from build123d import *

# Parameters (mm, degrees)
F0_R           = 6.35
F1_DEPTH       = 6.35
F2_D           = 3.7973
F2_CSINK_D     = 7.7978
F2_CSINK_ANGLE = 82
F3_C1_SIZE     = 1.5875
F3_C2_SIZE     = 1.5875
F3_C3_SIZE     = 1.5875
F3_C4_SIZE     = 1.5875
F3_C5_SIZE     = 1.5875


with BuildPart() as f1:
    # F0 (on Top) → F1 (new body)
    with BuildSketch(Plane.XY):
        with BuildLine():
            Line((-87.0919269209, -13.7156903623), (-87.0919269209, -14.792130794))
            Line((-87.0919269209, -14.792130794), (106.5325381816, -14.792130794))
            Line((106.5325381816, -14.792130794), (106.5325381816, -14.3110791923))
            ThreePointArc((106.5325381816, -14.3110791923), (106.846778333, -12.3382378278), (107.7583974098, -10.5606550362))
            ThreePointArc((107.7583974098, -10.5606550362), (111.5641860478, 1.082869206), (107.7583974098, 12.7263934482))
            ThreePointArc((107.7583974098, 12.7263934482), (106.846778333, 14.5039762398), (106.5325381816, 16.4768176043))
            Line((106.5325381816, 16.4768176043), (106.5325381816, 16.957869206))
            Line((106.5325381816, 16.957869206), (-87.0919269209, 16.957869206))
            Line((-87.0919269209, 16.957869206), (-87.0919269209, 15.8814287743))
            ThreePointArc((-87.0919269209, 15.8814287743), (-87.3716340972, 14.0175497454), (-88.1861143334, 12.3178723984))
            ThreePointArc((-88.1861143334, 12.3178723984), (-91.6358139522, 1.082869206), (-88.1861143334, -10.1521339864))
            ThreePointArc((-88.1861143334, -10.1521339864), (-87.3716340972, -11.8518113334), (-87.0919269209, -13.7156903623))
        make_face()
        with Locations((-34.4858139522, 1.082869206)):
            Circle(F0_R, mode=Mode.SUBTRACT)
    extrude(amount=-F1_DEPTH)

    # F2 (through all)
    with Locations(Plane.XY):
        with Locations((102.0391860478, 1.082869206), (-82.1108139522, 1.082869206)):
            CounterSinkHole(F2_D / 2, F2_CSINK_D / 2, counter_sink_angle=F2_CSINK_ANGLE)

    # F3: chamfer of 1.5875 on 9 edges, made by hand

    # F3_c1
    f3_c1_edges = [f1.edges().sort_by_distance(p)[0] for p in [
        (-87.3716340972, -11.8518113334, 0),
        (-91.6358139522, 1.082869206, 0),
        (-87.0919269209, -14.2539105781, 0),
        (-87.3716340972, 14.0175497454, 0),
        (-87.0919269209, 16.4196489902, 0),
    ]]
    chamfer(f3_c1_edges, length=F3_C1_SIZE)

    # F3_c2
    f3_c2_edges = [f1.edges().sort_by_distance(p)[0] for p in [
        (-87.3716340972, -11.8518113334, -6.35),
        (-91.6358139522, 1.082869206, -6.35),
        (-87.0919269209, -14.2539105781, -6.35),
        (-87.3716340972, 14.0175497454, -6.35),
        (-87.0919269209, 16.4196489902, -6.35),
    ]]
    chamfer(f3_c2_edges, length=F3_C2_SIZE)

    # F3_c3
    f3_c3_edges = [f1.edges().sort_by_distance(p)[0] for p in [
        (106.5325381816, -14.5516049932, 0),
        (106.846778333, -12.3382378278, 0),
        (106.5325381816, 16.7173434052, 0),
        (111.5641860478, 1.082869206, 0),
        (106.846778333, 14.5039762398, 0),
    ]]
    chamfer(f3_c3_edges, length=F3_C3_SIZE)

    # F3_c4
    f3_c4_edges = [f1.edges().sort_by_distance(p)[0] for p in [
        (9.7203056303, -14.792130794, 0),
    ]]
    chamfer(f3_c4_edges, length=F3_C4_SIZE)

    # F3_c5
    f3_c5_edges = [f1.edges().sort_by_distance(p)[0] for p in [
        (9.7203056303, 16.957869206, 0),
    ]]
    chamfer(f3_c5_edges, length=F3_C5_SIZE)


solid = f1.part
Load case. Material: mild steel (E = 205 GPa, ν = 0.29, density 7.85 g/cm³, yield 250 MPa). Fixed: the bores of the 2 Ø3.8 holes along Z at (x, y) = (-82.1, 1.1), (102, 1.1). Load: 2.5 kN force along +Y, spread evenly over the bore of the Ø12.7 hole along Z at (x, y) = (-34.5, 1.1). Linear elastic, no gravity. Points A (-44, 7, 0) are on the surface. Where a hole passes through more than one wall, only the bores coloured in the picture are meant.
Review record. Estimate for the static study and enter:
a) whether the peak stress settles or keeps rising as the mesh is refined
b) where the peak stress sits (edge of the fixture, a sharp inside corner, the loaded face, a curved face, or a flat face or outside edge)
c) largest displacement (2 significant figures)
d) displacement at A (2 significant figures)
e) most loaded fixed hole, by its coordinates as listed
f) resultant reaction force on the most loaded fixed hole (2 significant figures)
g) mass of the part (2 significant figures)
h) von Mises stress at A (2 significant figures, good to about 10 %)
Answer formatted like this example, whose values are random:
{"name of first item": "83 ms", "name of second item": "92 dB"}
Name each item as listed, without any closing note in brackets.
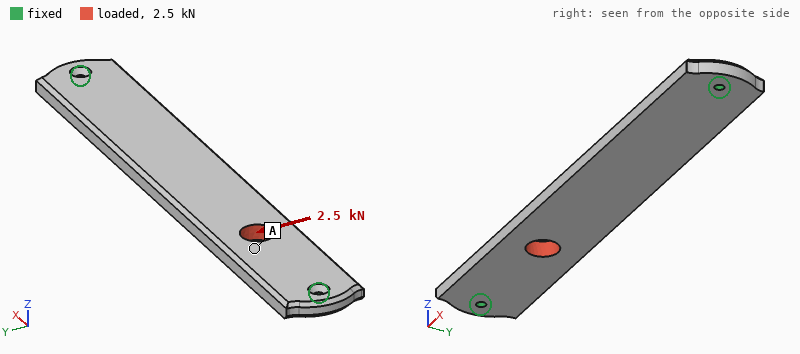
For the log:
{"whether the peak stress settles or keeps rising as the mesh is refined": "keeps rising", "where the peak stress sits": "edge of the fixture", "largest displacement": "59 µm", "displacement at A": "42 µm", "most loaded fixed hole, by its coordinates as listed": "(-82.1, 1.1)", "resultant reaction force on the most loaded fixed hole": "1.9 kN", "mass of the part": "300 g", "von Mises stress at A": "30 MPa"}
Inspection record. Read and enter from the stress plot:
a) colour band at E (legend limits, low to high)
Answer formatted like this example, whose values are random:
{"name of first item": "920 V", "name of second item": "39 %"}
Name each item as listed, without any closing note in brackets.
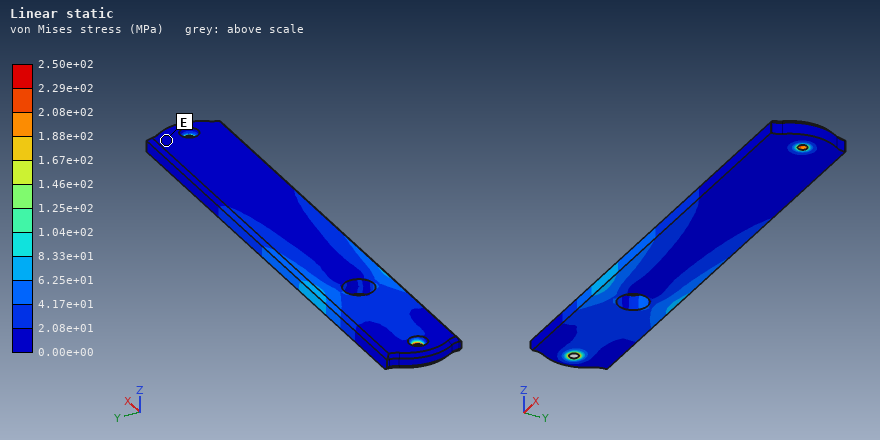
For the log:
{"colour band at E": "0.00e+00 to 2.08e+01 MPa"}
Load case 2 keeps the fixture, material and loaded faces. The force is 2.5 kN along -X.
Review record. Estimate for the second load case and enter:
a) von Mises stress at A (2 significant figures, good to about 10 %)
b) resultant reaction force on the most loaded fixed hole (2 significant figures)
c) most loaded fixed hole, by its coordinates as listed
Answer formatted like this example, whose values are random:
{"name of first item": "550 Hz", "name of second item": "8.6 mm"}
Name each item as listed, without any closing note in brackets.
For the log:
{"von Mises stress at A": "9.9 MPa", "resultant reaction force on the most loaded fixed hole": "1.7 kN", "most loaded fixed hole, by its coordinates as listed": "(-82.1, 1.1)"}
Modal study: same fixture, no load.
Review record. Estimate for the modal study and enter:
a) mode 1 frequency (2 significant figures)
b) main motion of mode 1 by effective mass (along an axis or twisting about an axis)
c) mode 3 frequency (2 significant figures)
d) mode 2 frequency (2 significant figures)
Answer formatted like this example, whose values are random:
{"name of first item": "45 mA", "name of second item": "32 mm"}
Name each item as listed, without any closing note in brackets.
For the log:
{"mode 1 frequency": "840 Hz", "main motion of mode 1 by effective mass": "along Z", "mode 3 frequency": "2400 Hz", "mode 2 frequency": "2300 Hz"}
